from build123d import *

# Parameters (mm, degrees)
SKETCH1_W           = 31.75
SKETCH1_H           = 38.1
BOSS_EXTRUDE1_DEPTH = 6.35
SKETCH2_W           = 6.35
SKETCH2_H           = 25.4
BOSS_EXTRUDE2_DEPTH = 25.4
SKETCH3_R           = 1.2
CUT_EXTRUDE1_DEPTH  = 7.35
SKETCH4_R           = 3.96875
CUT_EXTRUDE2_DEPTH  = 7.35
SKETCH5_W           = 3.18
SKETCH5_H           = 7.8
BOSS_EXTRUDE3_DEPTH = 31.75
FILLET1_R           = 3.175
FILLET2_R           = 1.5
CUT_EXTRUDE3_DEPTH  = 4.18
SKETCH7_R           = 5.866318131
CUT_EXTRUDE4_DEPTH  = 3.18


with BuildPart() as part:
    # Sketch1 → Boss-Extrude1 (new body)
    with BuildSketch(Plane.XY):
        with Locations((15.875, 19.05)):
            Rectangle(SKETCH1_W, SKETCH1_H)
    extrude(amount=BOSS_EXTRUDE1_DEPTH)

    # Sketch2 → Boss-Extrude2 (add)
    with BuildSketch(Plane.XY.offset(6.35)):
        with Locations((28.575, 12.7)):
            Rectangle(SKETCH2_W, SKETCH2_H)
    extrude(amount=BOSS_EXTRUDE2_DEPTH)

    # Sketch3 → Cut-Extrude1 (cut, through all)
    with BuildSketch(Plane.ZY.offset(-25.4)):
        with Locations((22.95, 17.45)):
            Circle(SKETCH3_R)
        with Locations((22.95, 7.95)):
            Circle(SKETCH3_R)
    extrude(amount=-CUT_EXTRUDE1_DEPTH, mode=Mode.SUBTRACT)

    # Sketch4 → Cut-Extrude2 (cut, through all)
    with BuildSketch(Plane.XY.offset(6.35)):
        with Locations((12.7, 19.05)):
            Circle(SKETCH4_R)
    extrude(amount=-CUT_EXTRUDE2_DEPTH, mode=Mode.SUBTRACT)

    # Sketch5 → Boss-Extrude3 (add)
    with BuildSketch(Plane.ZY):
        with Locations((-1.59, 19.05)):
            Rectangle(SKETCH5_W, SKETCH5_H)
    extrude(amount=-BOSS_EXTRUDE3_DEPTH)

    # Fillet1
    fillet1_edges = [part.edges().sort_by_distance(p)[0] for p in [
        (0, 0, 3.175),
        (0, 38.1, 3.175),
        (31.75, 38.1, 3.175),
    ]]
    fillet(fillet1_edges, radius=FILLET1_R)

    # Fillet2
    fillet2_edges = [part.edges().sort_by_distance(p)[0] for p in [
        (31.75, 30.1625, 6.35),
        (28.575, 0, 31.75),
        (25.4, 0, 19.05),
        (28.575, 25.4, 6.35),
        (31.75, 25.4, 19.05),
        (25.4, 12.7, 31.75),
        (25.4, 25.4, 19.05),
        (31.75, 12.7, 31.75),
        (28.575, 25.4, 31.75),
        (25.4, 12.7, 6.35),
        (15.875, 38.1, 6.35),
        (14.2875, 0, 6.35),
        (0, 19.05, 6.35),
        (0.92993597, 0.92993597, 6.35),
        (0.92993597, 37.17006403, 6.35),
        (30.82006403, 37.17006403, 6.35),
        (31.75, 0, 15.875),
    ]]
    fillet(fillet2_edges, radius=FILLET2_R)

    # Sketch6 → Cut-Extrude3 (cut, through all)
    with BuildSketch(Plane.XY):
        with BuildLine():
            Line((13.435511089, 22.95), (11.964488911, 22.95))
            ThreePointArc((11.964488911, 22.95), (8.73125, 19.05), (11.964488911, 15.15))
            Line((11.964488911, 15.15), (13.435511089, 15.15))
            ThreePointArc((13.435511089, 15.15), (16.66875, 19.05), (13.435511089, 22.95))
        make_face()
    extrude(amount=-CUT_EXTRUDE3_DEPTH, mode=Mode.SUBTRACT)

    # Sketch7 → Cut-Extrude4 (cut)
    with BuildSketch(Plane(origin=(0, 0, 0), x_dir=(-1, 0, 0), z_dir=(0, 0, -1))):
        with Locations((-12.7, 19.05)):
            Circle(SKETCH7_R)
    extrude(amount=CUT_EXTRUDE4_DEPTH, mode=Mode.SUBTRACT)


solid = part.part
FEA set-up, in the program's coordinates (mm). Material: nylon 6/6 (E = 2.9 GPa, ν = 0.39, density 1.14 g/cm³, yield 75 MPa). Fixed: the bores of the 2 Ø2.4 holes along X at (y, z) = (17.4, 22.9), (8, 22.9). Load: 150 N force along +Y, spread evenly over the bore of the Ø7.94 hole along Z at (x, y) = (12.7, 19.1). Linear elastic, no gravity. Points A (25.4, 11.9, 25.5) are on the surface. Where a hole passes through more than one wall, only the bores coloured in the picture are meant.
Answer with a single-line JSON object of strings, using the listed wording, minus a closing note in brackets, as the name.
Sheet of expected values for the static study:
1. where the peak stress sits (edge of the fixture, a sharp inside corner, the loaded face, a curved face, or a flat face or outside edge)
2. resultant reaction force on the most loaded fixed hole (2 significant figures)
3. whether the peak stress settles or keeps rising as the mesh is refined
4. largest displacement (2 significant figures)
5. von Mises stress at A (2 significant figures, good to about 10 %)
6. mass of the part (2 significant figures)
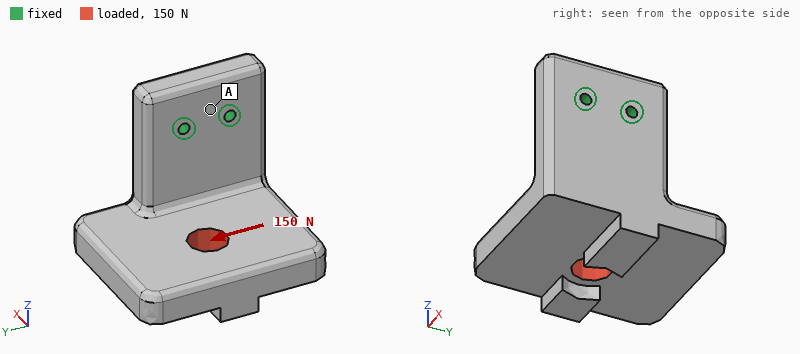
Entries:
{"where the peak stress sits": "edge of the fixture", "resultant reaction force on the most loaded fixed hole": "310 N", "whether the peak stress settles or keeps rising as the mesh is refined": "keeps rising", "largest displacement": "0.65 mm", "von Mises stress at A": "3.0 MPa", "mass of the part": "13 g"}
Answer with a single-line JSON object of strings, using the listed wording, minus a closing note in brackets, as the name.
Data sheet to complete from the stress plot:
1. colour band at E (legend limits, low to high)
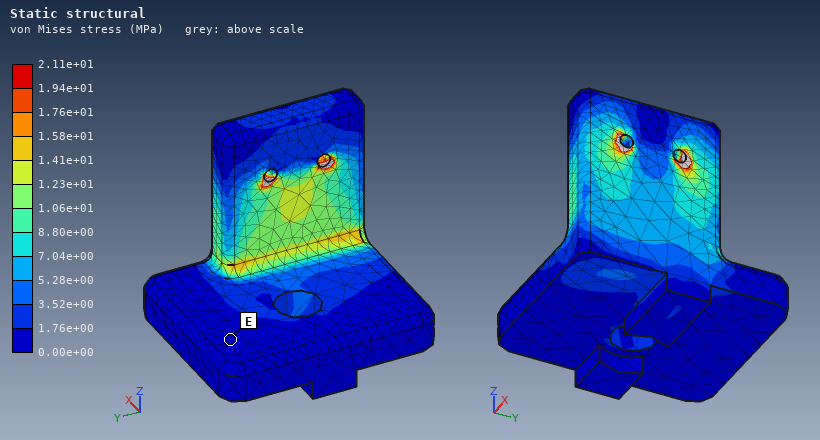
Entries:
{"colour band at E": "0.00e+00 to 1.76e+00 MPa"}
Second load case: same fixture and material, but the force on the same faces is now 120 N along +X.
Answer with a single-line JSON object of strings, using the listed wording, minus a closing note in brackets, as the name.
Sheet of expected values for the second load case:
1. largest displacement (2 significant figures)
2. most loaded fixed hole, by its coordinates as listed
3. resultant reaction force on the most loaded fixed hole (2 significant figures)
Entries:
{"largest displacement": "0.65 mm", "most loaded fixed hole, by its coordinates as listed": "(17.4, 22.9)", "resultant reaction force on the most loaded fixed hole": "110 N"}
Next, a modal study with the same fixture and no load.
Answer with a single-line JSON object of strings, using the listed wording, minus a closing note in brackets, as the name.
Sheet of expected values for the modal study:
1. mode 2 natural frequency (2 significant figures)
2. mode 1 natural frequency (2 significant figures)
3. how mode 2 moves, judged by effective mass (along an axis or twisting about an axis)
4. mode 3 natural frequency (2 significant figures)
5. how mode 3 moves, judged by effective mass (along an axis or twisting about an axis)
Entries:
{"mode 2 natural frequency": "1000 Hz", "mode 1 natural frequency": "720 Hz", "how mode 2 moves, judged by effective mass": "along Y", "mode 3 natural frequency": "2100 Hz", "how mode 3 moves, judged by effective mass": "along X"}
